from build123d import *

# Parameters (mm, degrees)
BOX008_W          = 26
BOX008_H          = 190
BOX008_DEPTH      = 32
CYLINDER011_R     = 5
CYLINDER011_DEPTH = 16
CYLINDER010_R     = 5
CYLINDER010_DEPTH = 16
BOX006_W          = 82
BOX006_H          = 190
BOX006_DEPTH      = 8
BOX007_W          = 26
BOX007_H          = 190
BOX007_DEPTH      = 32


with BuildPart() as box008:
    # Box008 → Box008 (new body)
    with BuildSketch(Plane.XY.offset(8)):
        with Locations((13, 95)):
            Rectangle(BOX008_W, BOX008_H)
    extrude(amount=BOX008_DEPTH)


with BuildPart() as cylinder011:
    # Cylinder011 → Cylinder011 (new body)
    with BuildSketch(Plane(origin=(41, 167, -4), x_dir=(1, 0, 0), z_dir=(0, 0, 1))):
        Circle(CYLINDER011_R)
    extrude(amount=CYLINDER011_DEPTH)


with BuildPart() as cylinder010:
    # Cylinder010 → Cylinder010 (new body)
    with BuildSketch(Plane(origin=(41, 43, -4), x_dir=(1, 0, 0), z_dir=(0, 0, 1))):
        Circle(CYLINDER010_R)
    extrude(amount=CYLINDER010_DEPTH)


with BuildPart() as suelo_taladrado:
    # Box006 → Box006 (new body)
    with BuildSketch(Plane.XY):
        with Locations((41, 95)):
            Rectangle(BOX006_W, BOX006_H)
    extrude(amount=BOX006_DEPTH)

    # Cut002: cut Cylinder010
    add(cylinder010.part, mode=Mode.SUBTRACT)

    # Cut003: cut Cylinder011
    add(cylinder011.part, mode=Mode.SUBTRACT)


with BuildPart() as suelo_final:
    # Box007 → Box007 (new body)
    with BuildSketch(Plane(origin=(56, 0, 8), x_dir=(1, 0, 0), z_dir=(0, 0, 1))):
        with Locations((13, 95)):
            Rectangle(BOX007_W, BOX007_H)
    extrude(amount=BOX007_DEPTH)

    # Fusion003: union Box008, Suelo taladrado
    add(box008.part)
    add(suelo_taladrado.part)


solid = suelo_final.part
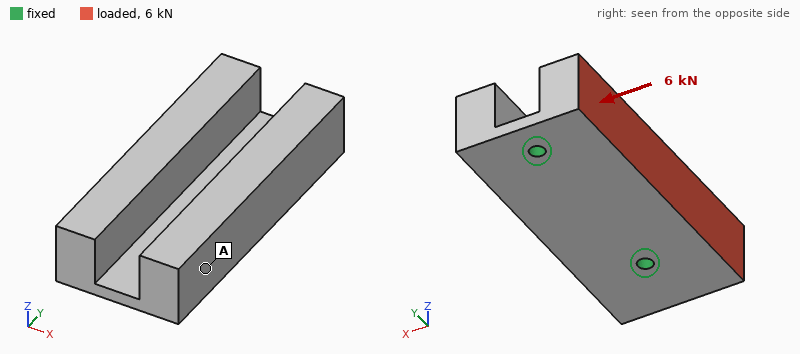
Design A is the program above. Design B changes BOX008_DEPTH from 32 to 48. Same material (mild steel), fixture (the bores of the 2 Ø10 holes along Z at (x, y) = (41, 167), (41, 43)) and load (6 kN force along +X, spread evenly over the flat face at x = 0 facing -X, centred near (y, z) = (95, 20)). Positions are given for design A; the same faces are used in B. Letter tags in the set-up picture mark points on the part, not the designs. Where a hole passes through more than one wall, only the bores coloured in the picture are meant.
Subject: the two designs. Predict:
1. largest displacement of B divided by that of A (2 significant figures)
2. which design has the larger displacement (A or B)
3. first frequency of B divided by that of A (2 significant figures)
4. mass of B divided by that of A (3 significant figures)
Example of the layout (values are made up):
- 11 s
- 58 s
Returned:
- 1.9
- B
- 0.77
- 1.18
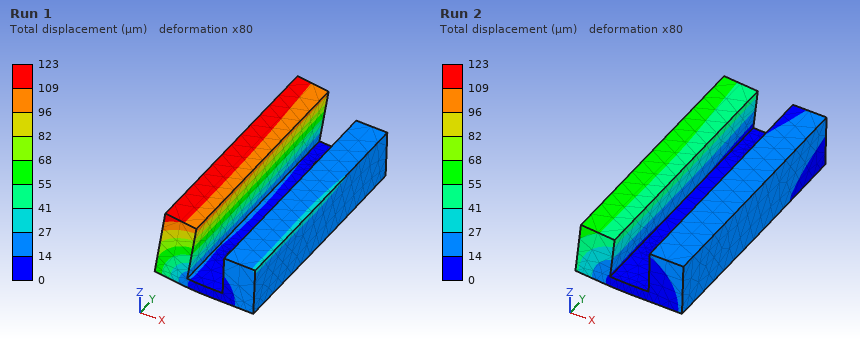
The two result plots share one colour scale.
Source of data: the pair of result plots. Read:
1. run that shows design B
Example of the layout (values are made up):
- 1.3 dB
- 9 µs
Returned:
- Run 1
